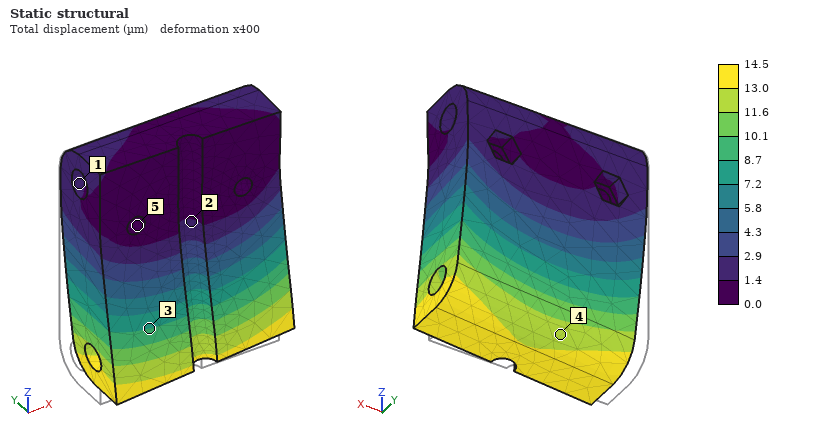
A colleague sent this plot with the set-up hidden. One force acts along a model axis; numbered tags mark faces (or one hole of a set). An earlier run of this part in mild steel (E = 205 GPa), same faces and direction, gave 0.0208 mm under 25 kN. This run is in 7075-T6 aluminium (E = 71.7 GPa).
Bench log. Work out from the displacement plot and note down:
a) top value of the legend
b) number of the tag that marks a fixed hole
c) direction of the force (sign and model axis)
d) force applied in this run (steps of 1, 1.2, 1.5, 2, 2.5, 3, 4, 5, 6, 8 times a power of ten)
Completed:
14.5 µm
5
+X
6 kN
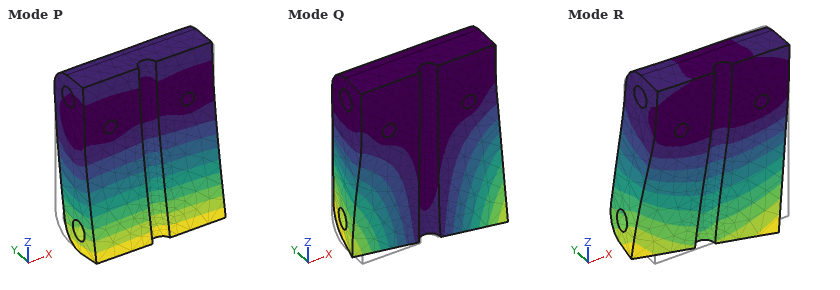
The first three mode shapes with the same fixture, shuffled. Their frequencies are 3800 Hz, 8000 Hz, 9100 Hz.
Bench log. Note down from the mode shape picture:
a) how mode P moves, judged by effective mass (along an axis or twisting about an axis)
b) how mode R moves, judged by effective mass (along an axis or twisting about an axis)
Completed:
along Y
along X
